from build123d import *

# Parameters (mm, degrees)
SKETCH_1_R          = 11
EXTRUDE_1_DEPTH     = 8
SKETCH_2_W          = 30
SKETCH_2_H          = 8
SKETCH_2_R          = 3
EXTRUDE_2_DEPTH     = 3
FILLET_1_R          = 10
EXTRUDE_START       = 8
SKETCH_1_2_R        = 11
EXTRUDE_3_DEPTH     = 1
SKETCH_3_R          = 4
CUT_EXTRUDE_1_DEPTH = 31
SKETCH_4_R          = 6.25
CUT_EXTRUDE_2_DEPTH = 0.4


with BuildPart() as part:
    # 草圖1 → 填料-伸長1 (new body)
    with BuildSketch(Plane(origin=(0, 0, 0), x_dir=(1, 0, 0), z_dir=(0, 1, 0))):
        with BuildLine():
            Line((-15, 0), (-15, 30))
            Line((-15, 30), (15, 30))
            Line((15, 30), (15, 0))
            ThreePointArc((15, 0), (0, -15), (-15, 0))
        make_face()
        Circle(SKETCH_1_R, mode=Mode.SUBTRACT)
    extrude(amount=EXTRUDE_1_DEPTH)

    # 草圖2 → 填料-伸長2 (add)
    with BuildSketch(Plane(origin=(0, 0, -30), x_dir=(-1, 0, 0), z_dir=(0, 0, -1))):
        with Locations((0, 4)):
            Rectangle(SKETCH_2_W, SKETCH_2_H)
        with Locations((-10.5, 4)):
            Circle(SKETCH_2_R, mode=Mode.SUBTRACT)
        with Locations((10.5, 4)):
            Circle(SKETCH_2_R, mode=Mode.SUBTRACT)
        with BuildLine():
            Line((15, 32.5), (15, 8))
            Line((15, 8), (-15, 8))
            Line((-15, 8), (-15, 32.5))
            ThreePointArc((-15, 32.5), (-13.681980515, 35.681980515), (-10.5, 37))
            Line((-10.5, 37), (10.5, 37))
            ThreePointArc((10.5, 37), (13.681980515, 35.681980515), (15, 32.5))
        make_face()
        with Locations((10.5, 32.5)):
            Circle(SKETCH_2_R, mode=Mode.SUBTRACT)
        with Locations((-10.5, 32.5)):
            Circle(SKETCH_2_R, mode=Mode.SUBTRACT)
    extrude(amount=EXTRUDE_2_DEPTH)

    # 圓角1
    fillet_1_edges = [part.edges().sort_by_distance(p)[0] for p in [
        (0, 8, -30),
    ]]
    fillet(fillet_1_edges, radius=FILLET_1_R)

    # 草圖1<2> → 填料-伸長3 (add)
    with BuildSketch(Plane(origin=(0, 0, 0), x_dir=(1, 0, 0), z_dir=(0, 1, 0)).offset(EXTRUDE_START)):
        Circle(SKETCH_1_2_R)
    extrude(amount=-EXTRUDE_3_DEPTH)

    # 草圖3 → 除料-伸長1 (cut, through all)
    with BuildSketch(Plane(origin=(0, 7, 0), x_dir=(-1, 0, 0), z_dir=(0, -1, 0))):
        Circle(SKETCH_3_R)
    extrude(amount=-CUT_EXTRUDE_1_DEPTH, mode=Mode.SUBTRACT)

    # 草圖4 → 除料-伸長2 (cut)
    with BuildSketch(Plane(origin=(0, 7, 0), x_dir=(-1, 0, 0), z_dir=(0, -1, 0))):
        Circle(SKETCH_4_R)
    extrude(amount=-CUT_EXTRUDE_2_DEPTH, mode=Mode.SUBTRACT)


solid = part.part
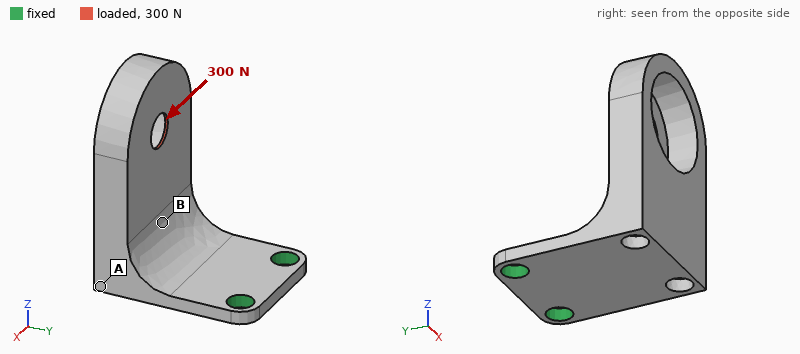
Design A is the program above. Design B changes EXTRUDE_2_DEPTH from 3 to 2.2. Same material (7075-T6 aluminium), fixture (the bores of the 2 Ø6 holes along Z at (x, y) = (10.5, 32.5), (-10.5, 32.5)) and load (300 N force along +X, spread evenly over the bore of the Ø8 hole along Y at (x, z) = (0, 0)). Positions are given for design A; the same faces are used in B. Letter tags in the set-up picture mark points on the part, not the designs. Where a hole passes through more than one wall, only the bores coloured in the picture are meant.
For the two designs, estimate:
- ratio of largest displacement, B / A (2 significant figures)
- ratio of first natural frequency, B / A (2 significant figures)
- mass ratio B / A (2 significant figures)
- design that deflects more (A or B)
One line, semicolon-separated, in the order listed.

2.0; 0.65; 0.93; B
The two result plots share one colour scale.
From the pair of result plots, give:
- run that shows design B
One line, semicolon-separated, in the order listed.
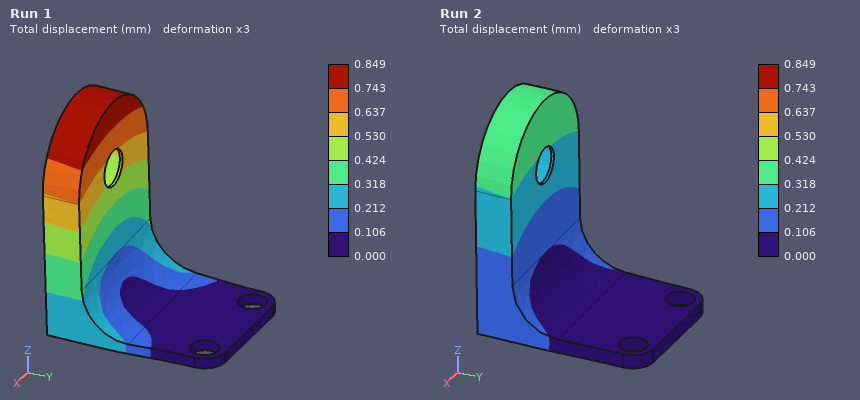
Run 1
